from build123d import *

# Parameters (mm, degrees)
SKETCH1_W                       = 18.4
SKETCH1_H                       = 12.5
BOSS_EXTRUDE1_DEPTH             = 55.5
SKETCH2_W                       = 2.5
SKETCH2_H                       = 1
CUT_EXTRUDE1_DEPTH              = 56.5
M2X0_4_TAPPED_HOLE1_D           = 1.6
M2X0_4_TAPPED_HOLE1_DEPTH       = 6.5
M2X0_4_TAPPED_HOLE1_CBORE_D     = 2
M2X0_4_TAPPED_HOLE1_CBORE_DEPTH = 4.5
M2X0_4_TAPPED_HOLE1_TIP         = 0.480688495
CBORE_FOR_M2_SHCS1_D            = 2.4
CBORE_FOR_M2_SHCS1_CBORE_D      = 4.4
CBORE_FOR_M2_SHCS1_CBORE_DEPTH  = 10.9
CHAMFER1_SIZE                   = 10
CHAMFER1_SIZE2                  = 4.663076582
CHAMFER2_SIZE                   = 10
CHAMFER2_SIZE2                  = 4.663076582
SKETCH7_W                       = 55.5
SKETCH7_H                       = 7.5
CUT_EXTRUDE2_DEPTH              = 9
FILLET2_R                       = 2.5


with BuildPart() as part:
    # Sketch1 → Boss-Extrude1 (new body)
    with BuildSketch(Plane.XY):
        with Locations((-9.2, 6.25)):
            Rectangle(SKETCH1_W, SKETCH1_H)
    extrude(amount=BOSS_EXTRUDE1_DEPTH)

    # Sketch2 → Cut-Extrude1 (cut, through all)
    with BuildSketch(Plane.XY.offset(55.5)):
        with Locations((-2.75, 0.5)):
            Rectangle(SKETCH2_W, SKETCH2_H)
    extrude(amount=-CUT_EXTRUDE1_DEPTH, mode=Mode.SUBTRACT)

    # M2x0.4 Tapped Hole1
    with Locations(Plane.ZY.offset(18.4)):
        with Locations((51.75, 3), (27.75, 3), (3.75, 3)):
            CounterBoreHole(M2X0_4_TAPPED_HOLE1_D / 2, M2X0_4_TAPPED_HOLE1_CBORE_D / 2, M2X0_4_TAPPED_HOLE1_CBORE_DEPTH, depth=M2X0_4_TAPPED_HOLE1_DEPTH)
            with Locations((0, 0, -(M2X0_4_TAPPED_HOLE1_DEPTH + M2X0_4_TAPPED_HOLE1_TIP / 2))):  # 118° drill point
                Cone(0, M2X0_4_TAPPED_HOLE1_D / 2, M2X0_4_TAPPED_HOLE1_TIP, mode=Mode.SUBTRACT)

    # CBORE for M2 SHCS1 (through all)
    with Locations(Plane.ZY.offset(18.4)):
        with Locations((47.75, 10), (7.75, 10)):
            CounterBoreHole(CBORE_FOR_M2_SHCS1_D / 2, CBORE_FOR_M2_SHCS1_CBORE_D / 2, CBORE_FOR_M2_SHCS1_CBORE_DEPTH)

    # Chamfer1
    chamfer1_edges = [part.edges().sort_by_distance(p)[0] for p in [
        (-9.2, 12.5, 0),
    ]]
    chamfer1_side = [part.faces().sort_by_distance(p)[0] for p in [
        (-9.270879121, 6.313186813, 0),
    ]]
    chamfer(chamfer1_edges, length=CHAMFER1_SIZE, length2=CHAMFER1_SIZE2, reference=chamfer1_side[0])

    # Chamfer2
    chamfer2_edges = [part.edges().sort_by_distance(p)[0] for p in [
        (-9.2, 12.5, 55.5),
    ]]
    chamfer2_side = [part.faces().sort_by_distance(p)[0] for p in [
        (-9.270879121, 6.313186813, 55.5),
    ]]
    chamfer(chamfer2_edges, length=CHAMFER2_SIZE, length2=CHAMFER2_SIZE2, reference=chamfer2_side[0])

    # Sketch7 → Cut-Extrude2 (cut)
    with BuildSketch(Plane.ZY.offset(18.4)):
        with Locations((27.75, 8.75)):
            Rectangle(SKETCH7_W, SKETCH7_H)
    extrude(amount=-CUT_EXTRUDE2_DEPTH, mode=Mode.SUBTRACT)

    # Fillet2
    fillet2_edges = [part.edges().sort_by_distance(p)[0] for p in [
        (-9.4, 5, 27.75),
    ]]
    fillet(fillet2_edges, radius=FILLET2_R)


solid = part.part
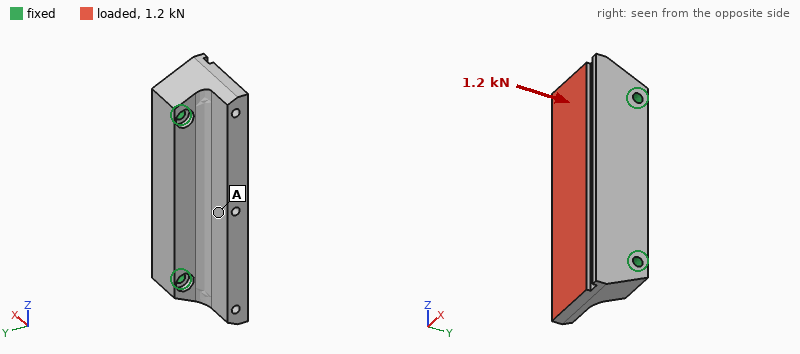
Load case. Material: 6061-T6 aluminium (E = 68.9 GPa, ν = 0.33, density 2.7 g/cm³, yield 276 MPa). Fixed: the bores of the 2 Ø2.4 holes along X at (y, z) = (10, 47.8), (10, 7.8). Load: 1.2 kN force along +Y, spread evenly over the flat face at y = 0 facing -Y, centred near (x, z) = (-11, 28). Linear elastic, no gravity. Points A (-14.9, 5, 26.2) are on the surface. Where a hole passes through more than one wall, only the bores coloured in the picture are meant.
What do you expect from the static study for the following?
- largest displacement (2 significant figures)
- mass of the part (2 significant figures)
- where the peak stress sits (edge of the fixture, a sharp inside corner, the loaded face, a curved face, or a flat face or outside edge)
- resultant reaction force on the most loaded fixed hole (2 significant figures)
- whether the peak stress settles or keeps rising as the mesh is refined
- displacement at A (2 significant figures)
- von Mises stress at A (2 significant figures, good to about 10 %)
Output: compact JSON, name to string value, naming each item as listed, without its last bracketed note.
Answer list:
{"largest displacement": "25 µm", "mass of the part": "22 g", "where the peak stress sits": "edge of the fixture", "resultant reaction force on the most loaded fixed hole": "650 N", "whether the peak stress settles or keeps rising as the mesh is refined": "keeps rising", "displacement at A": "18 µm", "von Mises stress at A": "7.6 MPa"}
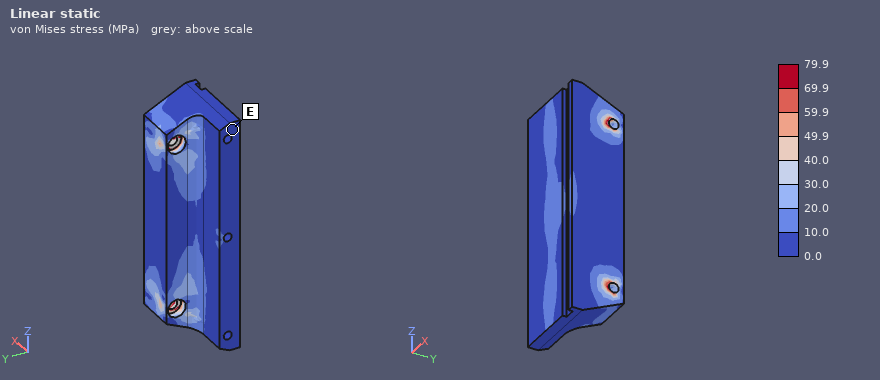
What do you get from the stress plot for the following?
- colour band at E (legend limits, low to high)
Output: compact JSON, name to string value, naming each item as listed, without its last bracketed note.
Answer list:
{"colour band at E": "0.0 to 10.0 MPa"}
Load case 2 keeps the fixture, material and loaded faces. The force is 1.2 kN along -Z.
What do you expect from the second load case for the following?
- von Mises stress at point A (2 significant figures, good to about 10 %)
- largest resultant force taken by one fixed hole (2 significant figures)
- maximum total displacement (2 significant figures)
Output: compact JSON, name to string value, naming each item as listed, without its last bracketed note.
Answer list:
{"von Mises stress at point A": "4.1 MPa", "largest resultant force taken by one fixed hole": "690 N", "maximum total displacement": "5.1 µm"}
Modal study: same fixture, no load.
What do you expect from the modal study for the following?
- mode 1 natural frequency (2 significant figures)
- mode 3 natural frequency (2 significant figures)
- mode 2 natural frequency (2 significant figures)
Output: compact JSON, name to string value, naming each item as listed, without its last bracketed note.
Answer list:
{"mode 1 natural frequency": "11 kHz", "mode 3 natural frequency": "20 kHz", "mode 2 natural frequency": "20 kHz"}
